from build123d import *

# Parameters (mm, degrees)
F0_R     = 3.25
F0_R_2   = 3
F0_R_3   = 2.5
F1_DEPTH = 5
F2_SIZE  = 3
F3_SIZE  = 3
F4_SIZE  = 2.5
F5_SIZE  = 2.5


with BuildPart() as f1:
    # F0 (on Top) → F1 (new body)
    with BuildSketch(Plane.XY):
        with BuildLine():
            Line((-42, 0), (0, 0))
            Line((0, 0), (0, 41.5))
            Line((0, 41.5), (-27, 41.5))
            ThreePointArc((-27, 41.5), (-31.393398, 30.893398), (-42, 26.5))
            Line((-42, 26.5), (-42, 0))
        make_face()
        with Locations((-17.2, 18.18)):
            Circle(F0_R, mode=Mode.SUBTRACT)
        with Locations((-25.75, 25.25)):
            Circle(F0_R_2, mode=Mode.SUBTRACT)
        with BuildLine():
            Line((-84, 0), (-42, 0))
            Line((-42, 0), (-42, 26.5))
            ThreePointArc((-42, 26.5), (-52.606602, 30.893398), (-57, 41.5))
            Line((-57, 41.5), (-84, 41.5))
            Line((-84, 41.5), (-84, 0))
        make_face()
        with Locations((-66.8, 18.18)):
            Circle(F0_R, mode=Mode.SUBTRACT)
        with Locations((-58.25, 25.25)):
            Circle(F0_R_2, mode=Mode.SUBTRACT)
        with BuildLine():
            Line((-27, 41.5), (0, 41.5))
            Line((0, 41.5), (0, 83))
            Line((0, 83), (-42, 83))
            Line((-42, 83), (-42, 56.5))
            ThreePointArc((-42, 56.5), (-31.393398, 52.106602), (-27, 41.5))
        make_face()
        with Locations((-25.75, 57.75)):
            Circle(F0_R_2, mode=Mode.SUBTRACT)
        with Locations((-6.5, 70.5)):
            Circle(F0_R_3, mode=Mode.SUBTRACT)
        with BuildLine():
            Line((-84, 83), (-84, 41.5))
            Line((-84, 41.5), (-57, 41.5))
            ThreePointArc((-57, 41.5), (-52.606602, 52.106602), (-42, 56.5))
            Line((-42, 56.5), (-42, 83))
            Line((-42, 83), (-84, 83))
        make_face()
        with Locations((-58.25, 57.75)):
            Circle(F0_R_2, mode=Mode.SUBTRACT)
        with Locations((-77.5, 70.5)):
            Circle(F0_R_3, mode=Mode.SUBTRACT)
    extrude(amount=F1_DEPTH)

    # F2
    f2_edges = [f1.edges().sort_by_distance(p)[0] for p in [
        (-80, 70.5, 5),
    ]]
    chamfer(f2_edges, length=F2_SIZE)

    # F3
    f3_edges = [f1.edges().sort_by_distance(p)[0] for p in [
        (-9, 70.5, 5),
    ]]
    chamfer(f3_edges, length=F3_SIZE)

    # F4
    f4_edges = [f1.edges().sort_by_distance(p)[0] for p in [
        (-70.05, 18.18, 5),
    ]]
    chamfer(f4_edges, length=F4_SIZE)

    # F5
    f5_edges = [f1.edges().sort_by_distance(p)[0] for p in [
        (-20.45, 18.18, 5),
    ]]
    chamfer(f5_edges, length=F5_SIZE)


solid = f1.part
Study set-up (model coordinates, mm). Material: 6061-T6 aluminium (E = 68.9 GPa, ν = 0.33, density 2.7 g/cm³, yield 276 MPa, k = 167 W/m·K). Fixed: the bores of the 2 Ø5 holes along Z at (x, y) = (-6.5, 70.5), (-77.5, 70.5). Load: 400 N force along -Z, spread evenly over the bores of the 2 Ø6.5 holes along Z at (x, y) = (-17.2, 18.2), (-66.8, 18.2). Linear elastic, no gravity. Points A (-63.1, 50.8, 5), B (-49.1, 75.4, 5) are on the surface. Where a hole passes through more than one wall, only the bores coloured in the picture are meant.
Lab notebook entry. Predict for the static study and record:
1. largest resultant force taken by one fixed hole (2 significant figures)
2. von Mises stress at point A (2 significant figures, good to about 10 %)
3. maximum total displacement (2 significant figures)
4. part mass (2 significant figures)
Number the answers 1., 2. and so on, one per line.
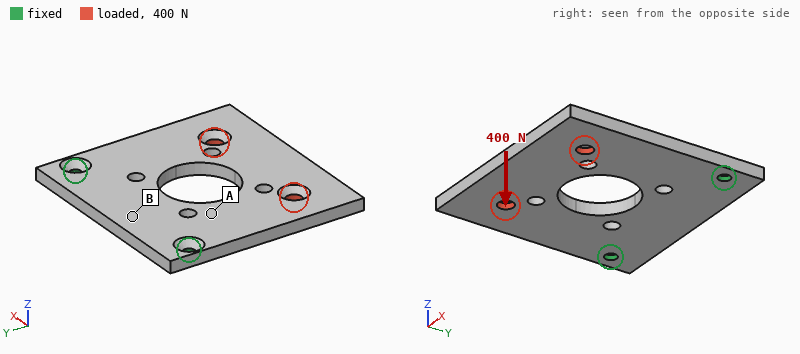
1. 290 N
2. 52 MPa
3. 1.2 mm
4. 81 g
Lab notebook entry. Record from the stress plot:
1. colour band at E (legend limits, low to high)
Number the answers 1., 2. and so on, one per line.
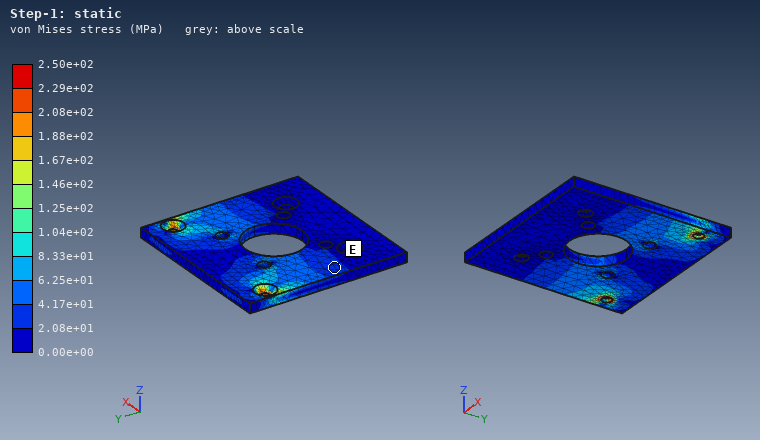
1. 2.08e+01 to 4.17e+01 MPa
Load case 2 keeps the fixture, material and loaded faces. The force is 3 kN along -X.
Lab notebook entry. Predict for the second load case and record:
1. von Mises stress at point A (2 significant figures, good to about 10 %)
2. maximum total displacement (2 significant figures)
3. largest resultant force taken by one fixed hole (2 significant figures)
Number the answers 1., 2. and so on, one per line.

1. 14 MPa
2. 0.15 mm
3. 2.6 kN
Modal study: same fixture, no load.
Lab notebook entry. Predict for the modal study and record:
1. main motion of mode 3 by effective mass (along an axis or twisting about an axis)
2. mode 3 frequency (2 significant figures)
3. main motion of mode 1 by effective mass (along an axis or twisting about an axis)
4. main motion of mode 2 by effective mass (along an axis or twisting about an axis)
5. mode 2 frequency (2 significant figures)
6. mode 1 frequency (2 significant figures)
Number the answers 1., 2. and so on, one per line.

1. along Z
2. 3500 Hz
3. along Z
4. twisting about Y
5. 1500 Hz
6. 540 Hz
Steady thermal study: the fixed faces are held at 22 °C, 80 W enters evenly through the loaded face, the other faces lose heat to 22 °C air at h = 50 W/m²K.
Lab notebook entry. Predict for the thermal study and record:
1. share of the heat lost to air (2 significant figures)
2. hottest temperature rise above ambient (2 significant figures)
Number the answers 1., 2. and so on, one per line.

1. 37 %
2. 82 K
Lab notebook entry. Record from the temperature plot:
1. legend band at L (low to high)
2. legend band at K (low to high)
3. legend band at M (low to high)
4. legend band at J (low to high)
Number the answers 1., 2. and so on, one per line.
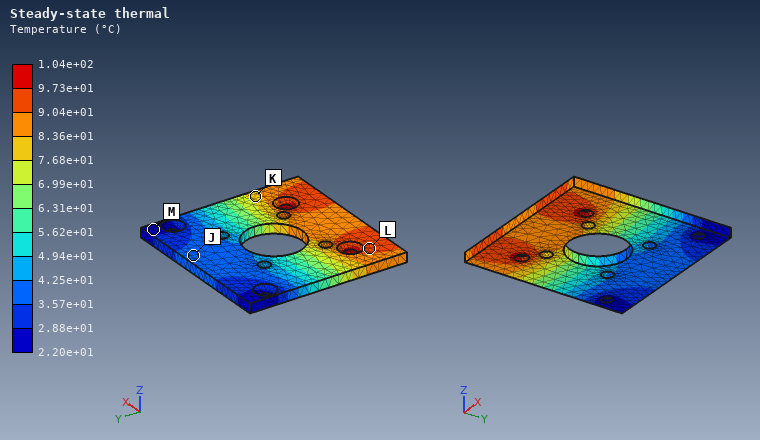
1. 9.04e+01 to 9.73e+01 °C
2. 7.68e+01 to 8.36e+01 °C
3. 2.20e+01 to 2.88e+01 °C
4. 3.57e+01 to 4.25e+01 °C
